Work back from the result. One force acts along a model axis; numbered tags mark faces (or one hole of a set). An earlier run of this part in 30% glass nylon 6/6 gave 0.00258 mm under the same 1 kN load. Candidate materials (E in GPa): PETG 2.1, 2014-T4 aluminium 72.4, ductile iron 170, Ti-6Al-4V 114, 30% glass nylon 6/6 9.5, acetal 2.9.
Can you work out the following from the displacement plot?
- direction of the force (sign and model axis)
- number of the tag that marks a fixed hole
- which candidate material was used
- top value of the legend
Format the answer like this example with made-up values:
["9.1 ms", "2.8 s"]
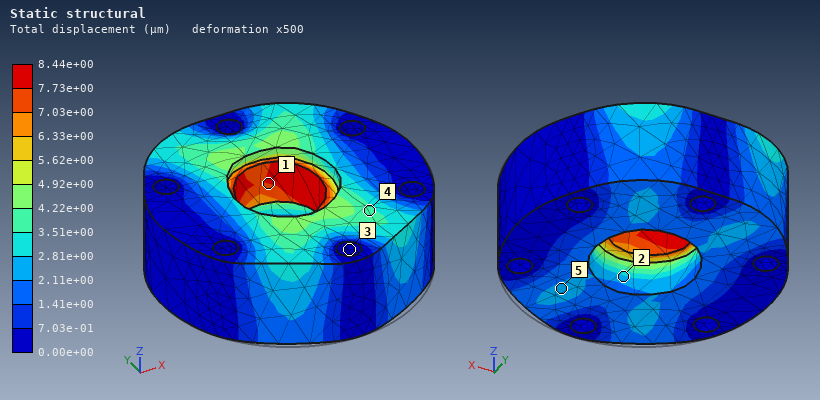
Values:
["+Y", "3", "acetal", "8.44e+00 µm"]
